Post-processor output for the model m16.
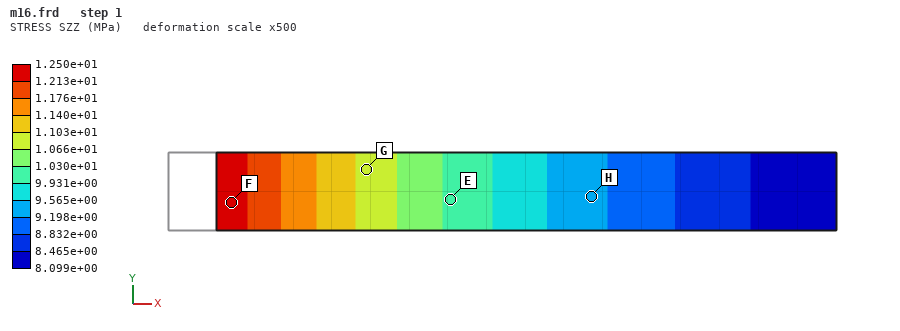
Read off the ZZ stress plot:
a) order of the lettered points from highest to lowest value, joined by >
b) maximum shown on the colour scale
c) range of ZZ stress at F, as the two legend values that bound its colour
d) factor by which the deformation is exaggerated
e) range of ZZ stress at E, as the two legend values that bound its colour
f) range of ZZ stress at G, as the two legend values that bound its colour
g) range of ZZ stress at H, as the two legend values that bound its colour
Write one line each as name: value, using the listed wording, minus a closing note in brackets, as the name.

order of the lettered points from highest to lowest value, joined by >: F > G > E > H
maximum shown on the colour scale: 1.250e+01 MPa
range of ZZ stress at F, as the two legend values that bound its colour: 1.213e+01 to 1.250e+01 MPa
factor by which the deformation is exaggerated: 500
range of ZZ stress at E, as the two legend values that bound its colour: 9.931e+00 to 1.030e+01 MPa
range of ZZ stress at G, as the two legend values that bound its colour: 1.066e+01 to 1.103e+01 MPa
range of ZZ stress at H, as the two legend values that bound its colour: 9.198e+00 to 9.565e+00 MPa
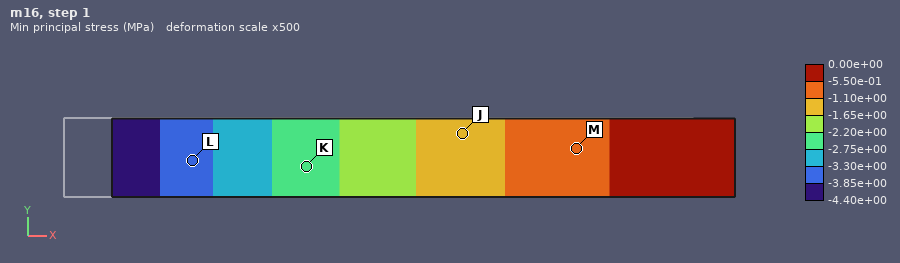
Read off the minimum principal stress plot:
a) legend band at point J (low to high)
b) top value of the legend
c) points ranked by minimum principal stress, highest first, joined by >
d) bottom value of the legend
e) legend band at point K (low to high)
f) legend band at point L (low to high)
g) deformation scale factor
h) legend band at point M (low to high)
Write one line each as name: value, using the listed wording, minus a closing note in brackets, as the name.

legend band at point J: -1.65e+00 to -1.10e+00 MPa
top value of the legend: 0.00e+00 MPa
points ranked by minimum principal stress, highest first, joined by >: M > J > K > L
bottom value of the legend: -4.40e+00 MPa
legend band at point K: -2.75e+00 to -2.20e+00 MPa
legend band at point L: -3.85e+00 to -3.30e+00 MPa
deformation scale factor: 500
legend band at point M: -1.10e+00 to -5.50e-01 MPa
